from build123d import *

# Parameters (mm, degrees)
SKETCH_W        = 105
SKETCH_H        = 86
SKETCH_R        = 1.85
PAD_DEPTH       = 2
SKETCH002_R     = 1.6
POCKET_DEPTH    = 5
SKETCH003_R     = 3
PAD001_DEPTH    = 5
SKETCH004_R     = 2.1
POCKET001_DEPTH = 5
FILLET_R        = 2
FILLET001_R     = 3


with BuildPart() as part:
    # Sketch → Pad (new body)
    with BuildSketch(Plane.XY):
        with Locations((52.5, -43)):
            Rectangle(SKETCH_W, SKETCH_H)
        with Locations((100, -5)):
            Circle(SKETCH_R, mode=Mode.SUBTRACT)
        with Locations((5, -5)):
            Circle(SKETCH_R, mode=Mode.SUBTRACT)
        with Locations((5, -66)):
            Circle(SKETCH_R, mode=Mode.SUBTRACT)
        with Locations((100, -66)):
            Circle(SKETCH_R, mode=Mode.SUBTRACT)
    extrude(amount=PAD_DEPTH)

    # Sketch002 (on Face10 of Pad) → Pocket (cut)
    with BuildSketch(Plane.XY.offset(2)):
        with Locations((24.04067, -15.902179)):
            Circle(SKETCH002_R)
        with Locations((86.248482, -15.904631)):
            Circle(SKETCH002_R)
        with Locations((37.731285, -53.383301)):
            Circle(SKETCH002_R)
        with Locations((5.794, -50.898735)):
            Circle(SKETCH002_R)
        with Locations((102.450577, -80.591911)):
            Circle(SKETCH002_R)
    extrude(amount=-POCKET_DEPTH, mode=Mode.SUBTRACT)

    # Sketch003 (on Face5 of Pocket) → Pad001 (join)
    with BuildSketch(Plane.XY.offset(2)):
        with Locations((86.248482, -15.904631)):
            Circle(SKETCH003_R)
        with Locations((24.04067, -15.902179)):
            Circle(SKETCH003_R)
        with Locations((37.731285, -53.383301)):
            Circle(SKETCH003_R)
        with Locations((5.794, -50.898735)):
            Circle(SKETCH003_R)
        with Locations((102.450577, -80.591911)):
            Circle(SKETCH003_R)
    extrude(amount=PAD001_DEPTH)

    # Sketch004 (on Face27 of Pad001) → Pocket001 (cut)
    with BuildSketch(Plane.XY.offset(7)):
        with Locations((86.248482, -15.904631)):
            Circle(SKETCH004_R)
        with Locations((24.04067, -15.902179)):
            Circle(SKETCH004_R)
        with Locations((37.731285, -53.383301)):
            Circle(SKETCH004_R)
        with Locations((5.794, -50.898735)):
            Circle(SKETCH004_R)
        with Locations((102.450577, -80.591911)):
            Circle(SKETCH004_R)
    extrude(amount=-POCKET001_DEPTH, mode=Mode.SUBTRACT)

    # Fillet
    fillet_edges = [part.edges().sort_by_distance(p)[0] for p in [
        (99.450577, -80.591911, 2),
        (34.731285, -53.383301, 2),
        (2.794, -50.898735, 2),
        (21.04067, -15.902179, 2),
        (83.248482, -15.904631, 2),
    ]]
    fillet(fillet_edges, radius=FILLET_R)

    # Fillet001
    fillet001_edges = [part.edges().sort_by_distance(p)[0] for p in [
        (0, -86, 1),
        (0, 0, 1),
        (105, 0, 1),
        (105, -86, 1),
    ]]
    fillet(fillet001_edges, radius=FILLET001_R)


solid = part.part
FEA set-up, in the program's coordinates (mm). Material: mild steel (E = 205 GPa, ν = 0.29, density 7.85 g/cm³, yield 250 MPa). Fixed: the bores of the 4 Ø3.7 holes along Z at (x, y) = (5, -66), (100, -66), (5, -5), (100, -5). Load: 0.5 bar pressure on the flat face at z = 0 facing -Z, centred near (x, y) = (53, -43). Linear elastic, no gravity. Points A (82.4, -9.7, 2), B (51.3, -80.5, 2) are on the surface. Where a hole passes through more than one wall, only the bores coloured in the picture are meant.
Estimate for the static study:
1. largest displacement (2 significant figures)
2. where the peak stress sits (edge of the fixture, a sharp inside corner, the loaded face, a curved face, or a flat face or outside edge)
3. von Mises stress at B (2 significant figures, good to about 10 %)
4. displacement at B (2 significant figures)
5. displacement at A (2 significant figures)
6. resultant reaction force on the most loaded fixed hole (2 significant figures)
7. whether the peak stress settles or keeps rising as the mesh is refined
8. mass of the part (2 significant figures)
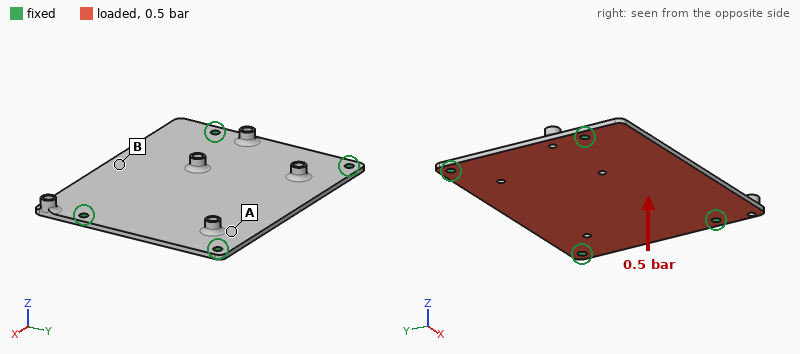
0.11 mm
edge of the fixture
34 MPa
0.11 mm
0.045 mm
130 N
keeps rising
140 g
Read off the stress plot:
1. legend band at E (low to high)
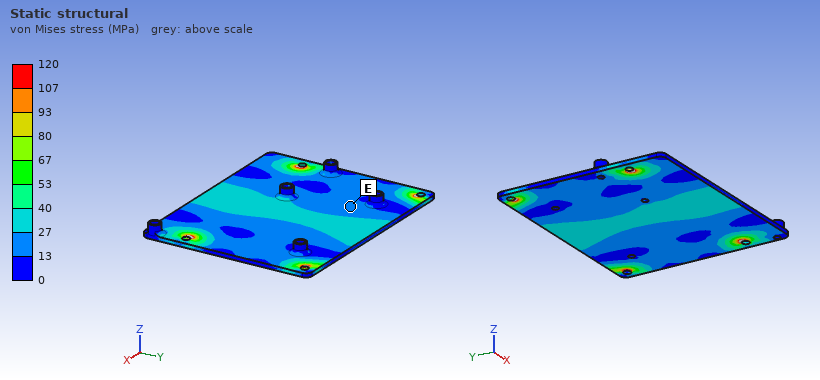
13 to 27 MPa
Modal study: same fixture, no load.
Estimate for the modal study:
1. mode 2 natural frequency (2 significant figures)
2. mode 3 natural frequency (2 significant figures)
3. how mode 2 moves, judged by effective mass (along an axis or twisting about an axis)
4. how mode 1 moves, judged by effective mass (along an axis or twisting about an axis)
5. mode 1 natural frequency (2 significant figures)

1300 Hz
2200 Hz
twisting about X
along Z
970 Hz
